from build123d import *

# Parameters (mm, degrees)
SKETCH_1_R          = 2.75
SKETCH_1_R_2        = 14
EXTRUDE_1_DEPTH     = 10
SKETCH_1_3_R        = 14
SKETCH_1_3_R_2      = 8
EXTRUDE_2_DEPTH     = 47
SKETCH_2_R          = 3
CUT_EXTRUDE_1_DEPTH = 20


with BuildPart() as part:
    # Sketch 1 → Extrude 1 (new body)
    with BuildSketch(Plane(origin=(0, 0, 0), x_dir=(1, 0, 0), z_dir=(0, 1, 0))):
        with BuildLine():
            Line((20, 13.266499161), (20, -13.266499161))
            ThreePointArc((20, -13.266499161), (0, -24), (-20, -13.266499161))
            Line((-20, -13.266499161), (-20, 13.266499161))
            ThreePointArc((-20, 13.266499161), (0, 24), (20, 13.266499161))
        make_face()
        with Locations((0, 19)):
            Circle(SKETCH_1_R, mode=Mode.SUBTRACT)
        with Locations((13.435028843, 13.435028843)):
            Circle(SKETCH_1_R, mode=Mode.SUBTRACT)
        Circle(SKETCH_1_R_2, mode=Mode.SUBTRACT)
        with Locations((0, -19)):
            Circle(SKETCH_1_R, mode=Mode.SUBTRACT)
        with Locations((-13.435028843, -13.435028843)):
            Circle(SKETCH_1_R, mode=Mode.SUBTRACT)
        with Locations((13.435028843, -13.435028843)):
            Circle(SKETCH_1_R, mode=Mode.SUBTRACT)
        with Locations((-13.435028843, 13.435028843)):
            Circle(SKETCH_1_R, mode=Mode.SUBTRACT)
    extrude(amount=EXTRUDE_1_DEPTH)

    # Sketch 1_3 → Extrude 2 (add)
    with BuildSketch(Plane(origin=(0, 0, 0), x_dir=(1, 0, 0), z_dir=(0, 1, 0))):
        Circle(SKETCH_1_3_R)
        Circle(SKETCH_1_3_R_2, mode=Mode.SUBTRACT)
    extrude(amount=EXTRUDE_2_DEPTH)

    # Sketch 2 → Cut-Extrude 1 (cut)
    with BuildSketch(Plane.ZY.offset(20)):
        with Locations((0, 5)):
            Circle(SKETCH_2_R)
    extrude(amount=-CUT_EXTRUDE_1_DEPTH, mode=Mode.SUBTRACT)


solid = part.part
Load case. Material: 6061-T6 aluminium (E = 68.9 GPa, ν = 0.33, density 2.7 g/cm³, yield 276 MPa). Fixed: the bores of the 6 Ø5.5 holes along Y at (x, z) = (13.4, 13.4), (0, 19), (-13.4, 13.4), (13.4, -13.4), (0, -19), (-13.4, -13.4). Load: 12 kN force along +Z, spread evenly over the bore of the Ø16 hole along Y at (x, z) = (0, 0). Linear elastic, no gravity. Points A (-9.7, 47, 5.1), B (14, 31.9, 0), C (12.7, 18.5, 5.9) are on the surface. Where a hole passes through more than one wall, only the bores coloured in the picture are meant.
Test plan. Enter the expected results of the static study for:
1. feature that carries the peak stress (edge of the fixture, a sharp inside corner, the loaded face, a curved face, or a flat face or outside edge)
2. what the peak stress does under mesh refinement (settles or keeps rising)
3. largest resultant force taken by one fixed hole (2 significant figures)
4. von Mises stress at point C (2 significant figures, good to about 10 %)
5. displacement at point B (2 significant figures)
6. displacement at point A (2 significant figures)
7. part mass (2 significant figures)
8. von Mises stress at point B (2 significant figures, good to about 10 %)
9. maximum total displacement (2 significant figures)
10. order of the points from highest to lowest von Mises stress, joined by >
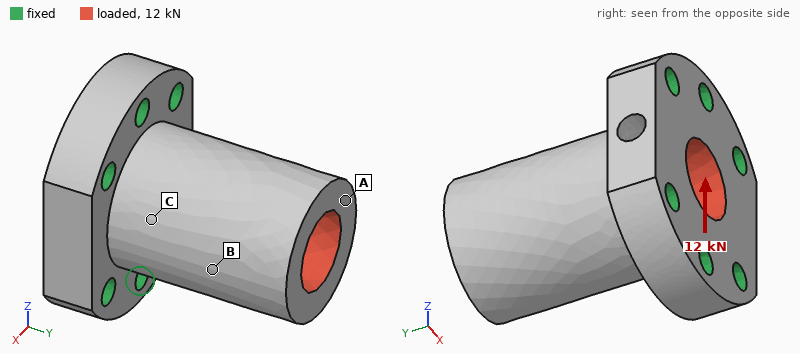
a sharp inside corner
keeps rising
4.3 kN
42 MPa
51 µm
83 µm
76 g
27 MPa
88 µm
C > B > A
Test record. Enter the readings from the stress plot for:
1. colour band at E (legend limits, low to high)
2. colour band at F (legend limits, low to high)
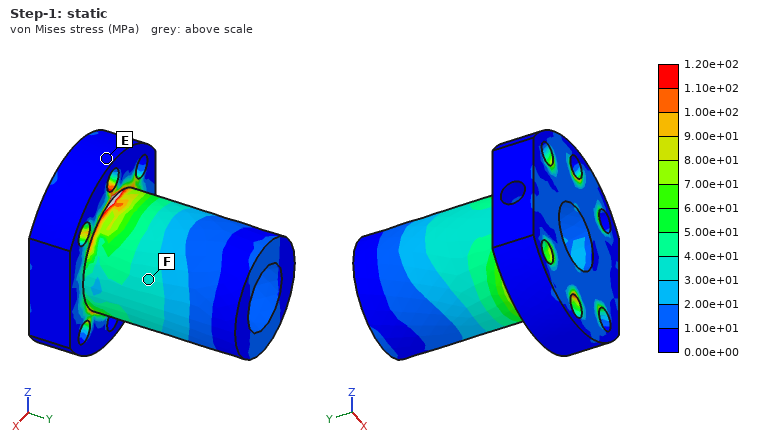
0.00e+00 to 1.00e+01 MPa
3.00e+01 to 4.00e+01 MPa
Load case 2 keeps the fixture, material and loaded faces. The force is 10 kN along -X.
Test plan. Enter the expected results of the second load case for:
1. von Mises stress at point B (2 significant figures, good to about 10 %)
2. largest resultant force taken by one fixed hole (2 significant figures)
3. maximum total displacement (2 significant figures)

14 MPa
4.2 kN
87 µm
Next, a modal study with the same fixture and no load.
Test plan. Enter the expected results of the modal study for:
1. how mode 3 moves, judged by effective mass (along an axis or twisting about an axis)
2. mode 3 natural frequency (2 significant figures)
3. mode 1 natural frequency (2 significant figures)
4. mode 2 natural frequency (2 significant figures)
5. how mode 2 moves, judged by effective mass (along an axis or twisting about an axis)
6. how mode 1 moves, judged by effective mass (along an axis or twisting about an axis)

twisting about Y
19 kHz
8900 Hz
9700 Hz
along Z
along X
